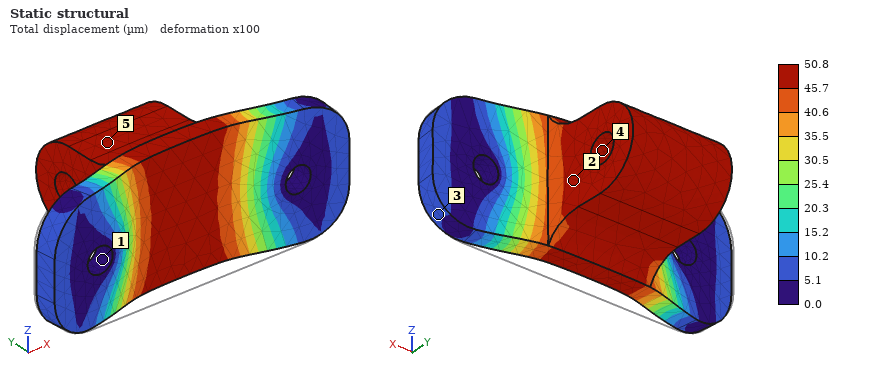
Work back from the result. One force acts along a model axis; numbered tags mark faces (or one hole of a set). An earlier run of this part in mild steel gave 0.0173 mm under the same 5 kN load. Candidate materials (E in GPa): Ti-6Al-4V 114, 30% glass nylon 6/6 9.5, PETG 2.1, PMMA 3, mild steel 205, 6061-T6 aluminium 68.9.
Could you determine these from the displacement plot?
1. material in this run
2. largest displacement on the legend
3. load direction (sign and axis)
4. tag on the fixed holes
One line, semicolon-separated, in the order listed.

6061-T6 aluminium; 50.8 µm; +Y; 1
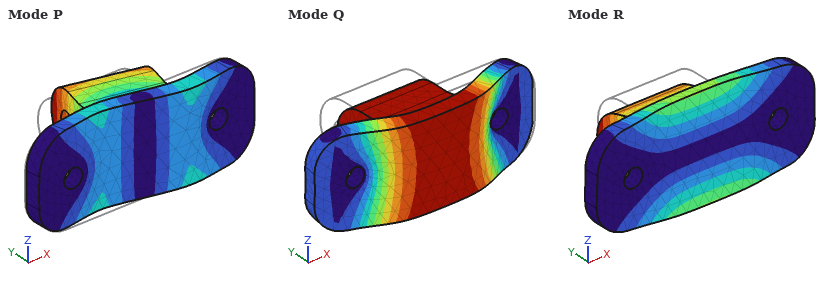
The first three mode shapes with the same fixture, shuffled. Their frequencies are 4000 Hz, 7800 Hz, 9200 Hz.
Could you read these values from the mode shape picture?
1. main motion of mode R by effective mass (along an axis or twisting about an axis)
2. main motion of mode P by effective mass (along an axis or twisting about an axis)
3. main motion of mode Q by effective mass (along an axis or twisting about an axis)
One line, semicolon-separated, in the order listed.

along Z; along X; along Y
